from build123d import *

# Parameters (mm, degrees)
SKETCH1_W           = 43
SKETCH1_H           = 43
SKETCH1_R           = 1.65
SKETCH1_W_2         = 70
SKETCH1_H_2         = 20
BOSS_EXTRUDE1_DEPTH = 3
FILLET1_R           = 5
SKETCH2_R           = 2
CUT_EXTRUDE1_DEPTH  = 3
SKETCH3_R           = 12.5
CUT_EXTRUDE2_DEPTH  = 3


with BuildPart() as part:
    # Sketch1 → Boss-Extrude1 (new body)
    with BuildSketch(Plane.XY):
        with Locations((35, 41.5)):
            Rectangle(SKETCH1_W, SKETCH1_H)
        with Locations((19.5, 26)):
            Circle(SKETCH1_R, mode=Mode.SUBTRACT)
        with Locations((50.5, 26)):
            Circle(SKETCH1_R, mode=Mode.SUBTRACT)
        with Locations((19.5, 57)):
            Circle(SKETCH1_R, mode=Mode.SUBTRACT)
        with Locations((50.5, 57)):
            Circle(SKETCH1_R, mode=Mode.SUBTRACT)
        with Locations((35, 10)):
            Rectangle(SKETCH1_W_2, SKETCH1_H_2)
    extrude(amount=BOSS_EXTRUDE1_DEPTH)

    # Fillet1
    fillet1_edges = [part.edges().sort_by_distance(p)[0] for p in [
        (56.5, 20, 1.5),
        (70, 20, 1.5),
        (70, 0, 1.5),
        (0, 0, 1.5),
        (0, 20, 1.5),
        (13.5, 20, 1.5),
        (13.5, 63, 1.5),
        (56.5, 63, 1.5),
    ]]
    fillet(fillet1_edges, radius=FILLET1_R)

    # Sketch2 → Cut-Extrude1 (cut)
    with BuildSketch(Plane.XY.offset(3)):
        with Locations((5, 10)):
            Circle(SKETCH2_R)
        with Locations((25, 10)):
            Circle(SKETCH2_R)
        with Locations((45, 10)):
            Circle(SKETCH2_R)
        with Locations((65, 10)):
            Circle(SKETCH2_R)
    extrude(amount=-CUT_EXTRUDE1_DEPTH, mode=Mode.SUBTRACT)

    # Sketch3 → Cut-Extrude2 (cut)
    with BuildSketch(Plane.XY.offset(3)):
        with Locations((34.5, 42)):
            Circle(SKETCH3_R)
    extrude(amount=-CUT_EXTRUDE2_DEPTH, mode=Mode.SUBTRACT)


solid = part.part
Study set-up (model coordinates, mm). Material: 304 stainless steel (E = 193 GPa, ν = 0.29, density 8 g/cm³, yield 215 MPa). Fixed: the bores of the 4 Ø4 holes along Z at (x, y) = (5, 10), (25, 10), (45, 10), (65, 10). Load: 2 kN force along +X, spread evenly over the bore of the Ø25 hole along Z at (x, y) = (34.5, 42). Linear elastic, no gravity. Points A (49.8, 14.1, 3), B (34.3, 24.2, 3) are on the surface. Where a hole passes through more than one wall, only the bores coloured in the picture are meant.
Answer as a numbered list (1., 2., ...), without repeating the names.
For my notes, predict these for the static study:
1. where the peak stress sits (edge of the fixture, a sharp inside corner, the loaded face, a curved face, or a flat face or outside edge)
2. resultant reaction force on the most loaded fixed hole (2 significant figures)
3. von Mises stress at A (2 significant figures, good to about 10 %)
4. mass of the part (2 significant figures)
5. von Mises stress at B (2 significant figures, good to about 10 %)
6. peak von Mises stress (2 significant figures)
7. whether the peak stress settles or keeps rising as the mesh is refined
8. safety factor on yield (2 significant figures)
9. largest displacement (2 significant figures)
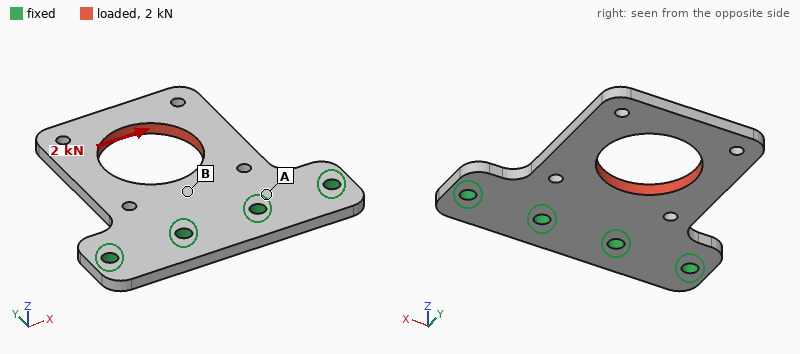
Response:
1. a curved face
2. 940 N
3. 14 MPa
4. 64 g
5. 55 MPa
6. 130 MPa
7. settles
8. 1.6
9. 38 µm
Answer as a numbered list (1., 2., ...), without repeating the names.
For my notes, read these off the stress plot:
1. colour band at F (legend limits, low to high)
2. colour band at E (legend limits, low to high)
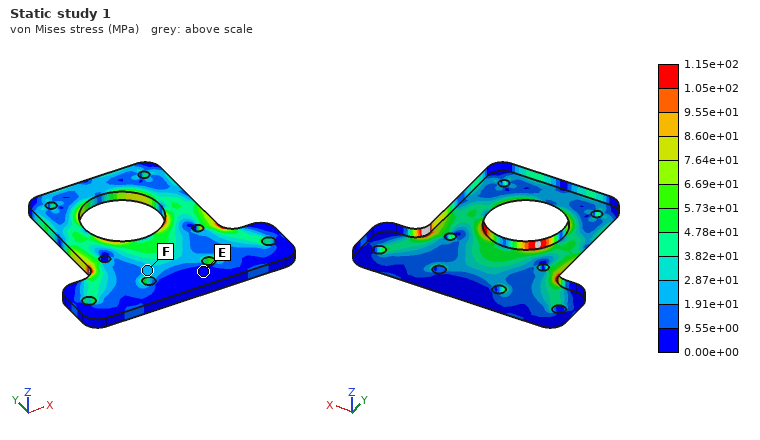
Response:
1. 1.91e+01 to 2.87e+01 MPa
2. 0.00e+00 to 9.55e+00 MPa
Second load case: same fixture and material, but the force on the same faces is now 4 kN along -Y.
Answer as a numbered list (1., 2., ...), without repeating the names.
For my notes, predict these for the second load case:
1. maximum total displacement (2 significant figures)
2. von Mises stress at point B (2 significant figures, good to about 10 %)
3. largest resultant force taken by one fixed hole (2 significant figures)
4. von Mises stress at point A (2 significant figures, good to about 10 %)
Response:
1. 17 µm
2. 14 MPa
3. 1.5 kN
4. 25 MPa
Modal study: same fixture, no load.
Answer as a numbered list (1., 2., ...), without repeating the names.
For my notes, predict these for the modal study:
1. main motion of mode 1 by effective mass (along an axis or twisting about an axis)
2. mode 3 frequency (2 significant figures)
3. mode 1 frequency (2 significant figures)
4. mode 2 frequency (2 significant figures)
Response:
1. along Z
2. 5100 Hz
3. 930 Hz
4. 2300 Hz
